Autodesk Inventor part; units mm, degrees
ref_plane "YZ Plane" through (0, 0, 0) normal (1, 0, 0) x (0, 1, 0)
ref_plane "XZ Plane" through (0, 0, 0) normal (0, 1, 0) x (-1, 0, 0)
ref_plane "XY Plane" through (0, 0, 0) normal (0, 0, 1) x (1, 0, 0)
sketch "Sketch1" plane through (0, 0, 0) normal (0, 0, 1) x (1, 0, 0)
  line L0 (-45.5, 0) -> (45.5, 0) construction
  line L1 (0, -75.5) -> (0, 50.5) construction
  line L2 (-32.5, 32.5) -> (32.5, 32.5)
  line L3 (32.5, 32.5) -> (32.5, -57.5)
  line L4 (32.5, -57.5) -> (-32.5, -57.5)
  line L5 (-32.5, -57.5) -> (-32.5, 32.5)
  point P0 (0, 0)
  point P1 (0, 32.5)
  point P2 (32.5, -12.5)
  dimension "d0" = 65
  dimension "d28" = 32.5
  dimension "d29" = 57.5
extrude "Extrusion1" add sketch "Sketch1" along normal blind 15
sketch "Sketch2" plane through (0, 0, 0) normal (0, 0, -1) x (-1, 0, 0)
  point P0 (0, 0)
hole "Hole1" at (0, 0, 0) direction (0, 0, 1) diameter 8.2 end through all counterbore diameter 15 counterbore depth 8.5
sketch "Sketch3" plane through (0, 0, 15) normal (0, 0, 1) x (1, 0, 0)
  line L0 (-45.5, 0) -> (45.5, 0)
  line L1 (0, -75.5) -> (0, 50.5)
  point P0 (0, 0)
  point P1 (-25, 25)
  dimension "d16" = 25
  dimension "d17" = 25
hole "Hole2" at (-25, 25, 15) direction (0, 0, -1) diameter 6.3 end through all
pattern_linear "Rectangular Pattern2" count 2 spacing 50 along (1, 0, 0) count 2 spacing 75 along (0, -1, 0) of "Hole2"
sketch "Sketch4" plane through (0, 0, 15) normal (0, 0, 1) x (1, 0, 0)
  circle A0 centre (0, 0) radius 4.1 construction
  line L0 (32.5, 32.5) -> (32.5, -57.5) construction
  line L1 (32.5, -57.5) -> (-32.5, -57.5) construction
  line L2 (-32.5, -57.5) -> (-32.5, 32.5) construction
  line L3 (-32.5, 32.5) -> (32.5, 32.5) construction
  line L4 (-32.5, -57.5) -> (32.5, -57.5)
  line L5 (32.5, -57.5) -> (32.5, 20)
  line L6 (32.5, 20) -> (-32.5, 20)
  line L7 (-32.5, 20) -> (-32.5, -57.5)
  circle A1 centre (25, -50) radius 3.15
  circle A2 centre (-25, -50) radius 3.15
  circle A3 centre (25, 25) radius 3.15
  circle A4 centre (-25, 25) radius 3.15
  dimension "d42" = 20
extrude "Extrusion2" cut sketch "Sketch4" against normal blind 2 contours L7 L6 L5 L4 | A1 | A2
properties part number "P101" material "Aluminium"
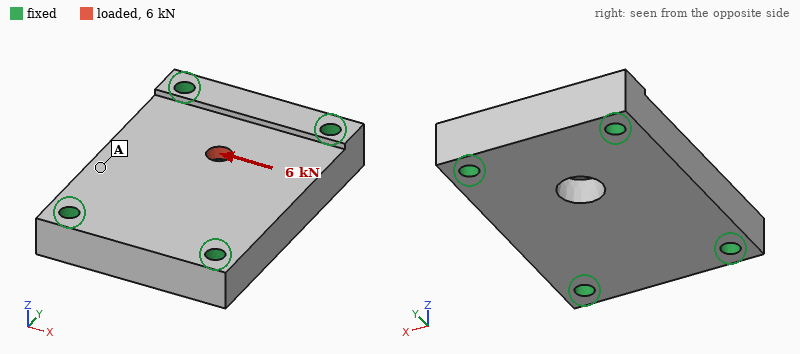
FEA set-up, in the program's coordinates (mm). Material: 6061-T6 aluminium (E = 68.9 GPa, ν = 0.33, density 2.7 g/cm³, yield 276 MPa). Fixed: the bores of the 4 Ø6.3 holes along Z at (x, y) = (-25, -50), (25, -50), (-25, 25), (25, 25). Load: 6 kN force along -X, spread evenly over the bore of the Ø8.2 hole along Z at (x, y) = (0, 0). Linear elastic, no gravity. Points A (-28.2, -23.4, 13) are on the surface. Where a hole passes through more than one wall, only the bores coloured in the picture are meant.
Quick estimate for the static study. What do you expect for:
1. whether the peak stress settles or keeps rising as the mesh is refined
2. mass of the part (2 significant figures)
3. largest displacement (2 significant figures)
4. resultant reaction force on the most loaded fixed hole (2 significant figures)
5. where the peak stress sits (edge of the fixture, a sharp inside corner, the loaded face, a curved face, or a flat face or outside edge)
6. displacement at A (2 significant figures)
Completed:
keeps rising
200 g
12 µm
2.3 kN
a sharp inside corner
4.6 µm
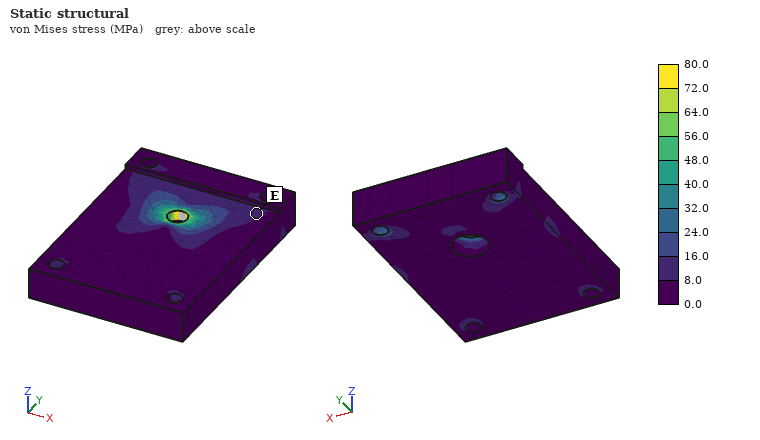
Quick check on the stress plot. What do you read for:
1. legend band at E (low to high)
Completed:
8.0 to 16.0 MPa
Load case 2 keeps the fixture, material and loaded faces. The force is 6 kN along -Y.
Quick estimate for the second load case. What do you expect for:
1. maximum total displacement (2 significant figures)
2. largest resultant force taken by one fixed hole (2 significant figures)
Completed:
11 µm
2.0 kN
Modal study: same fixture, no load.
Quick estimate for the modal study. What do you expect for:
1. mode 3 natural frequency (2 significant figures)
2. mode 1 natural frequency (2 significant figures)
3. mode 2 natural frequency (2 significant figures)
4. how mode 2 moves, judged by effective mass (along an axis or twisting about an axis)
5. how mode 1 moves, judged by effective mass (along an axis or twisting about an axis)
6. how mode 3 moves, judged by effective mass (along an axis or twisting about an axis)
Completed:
17 kHz
9000 Hz
12 kHz
twisting about Y
along Z
along X
